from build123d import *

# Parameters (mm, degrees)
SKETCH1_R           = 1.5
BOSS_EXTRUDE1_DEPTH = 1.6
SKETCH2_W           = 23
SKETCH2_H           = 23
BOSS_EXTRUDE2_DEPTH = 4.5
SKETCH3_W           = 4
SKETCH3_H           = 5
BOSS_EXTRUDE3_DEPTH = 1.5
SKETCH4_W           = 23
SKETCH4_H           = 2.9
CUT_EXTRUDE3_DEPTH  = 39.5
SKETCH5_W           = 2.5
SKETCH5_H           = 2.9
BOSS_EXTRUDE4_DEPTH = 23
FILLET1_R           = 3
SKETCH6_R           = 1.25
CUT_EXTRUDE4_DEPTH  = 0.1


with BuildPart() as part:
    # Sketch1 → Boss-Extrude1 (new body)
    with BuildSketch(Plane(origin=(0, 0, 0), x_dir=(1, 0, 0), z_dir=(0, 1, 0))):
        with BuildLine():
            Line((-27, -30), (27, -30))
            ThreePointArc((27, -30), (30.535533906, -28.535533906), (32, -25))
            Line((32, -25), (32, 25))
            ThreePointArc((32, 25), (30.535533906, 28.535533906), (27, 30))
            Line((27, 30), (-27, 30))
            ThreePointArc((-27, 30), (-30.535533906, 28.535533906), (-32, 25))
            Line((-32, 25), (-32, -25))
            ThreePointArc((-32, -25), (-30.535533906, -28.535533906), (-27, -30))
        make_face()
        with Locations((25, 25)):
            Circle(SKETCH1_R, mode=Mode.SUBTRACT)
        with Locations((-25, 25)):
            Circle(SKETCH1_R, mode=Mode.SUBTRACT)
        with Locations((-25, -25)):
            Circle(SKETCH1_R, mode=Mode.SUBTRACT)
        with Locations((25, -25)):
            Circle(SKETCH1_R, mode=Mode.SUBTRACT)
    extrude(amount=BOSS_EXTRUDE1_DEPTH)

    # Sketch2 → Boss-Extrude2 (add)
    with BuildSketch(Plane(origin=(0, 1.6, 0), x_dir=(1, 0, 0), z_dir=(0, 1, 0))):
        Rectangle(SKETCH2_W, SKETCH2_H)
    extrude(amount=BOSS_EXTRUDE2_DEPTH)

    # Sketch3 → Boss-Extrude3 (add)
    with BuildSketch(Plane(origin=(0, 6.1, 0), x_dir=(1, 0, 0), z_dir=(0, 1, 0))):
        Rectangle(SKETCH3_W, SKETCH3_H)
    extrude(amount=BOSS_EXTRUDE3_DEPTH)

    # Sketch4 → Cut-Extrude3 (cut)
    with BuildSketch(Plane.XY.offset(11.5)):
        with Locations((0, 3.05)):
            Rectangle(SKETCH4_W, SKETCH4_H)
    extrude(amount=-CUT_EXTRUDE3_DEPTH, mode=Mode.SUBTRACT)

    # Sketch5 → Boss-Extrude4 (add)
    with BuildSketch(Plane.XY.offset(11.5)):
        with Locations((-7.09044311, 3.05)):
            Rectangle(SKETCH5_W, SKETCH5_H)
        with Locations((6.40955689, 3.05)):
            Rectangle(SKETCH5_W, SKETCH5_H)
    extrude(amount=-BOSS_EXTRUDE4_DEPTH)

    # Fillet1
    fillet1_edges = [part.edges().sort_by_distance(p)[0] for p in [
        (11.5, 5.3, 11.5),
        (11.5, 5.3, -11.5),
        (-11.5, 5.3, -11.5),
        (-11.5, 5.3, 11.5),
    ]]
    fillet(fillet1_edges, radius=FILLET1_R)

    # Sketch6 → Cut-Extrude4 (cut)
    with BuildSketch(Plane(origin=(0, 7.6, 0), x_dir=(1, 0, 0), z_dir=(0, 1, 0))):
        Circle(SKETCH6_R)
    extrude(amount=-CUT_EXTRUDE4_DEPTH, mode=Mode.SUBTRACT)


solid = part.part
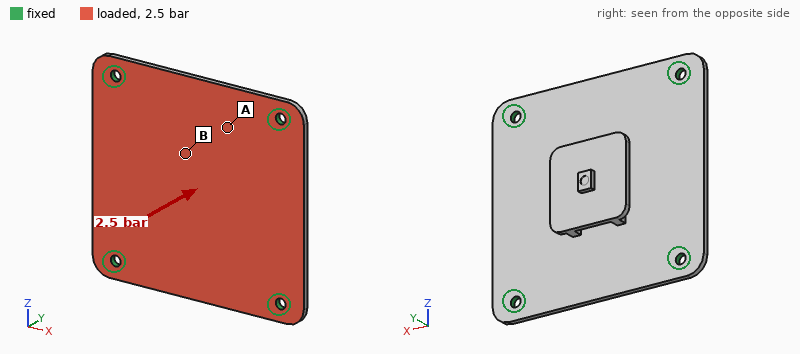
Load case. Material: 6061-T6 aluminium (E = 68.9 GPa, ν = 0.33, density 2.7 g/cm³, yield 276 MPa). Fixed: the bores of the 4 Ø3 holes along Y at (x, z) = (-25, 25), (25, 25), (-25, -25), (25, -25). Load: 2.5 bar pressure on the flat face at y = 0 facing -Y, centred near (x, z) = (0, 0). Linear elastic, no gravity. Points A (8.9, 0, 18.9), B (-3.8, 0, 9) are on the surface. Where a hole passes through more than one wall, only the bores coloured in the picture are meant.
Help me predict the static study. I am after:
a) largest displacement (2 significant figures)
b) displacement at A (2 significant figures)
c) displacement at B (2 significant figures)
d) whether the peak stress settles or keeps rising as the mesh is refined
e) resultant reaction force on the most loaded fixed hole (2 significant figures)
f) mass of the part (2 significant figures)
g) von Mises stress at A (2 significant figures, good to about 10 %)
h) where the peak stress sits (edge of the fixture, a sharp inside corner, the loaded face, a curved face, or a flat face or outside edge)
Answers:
0.27 mm
0.21 mm
0.27 mm
keeps rising
240 N
20 g
59 MPa
edge of the fixture
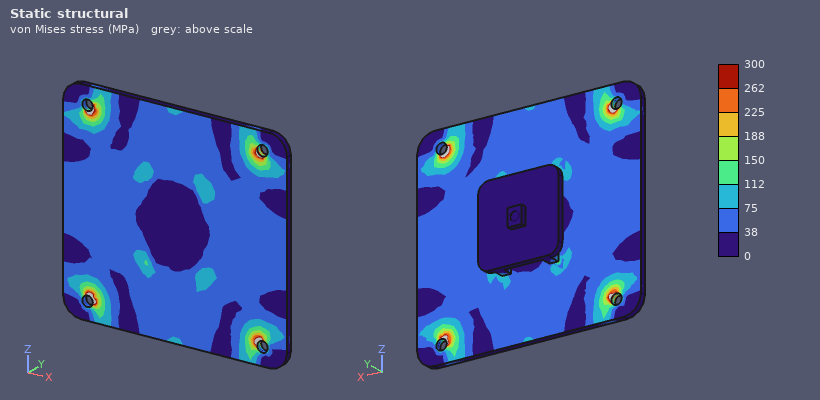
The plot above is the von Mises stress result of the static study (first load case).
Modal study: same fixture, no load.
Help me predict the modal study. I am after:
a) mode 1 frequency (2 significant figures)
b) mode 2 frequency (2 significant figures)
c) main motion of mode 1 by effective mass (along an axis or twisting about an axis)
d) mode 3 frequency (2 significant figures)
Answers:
2200 Hz
3700 Hz
along Y
3700 Hz
